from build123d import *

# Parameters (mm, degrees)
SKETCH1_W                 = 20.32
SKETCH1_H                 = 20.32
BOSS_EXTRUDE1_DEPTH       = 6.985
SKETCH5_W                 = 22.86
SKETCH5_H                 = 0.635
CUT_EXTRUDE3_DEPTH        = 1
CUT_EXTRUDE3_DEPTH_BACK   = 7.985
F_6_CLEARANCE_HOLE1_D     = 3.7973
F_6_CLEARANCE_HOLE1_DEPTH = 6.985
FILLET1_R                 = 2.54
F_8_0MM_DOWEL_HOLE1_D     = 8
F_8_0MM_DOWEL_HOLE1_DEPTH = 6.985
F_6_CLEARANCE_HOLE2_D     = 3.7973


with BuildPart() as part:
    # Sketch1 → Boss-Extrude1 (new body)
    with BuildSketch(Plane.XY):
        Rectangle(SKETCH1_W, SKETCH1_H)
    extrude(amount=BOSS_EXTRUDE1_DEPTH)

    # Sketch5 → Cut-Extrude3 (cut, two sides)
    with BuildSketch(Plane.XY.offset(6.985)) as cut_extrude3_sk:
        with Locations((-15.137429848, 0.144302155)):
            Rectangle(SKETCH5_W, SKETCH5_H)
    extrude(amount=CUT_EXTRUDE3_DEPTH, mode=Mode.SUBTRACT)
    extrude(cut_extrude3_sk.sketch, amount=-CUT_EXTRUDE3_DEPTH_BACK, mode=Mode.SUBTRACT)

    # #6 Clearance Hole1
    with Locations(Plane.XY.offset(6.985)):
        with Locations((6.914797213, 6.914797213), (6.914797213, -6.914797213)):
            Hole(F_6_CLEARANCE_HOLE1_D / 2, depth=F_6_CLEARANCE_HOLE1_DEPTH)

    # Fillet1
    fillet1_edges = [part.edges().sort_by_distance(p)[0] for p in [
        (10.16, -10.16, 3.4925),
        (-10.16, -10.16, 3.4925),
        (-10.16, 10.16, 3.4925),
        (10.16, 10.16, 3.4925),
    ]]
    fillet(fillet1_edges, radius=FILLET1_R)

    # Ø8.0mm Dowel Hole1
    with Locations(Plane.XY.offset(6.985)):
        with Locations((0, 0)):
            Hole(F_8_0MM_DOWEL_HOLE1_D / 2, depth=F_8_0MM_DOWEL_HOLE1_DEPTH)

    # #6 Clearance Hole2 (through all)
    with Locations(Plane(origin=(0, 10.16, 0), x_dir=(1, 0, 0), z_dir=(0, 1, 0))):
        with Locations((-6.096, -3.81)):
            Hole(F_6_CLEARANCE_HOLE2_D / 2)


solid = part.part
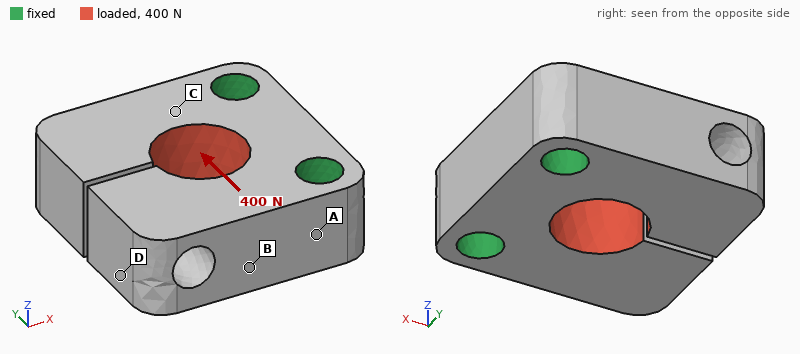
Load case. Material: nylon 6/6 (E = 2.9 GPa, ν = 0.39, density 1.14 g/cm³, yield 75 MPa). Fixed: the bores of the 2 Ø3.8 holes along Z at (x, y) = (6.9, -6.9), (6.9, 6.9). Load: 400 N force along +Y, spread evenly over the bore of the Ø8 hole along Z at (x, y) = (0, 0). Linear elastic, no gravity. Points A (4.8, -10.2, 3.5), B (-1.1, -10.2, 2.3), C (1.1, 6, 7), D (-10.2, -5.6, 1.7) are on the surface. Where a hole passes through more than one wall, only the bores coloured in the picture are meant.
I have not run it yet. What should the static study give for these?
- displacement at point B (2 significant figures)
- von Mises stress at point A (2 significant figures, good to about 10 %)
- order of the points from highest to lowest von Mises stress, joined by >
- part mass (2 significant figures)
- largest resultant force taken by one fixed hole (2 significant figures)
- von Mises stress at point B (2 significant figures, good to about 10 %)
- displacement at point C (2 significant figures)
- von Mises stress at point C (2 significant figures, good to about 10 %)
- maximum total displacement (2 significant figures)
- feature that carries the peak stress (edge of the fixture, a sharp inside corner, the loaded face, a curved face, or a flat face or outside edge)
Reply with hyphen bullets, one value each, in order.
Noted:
- 0.054 mm
- 9.9 MPa
- A > C > B > D
- 2.4 g
- 230 N
- 3.0 MPa
- 0.025 mm
- 6.4 MPa
- 0.13 mm
- the loaded face
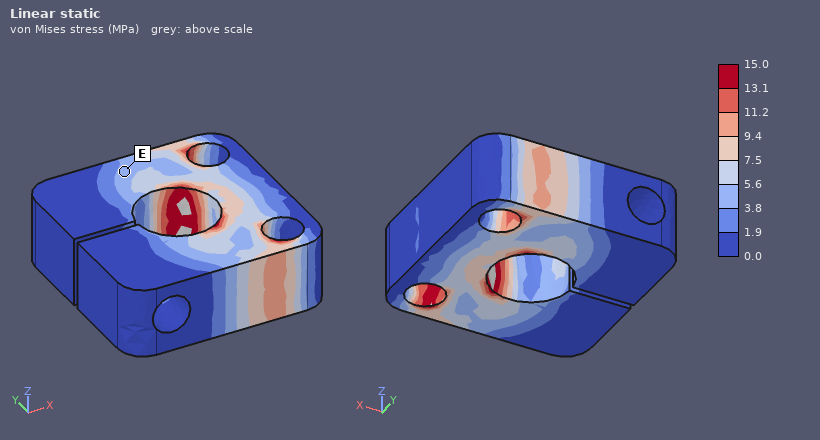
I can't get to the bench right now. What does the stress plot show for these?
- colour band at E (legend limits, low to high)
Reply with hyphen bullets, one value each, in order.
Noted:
- 3.8 to 5.6 MPa
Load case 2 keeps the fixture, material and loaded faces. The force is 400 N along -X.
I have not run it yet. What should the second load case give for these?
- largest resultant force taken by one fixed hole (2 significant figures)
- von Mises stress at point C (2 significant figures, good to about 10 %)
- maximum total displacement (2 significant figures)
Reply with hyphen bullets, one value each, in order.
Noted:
- 210 N
- 3.8 MPa
- 0.15 mm
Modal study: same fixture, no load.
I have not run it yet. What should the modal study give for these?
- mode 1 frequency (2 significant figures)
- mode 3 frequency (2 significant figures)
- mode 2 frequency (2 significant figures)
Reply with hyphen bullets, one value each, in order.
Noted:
- 5400 Hz
- 5600 Hz
- 5600 Hz
